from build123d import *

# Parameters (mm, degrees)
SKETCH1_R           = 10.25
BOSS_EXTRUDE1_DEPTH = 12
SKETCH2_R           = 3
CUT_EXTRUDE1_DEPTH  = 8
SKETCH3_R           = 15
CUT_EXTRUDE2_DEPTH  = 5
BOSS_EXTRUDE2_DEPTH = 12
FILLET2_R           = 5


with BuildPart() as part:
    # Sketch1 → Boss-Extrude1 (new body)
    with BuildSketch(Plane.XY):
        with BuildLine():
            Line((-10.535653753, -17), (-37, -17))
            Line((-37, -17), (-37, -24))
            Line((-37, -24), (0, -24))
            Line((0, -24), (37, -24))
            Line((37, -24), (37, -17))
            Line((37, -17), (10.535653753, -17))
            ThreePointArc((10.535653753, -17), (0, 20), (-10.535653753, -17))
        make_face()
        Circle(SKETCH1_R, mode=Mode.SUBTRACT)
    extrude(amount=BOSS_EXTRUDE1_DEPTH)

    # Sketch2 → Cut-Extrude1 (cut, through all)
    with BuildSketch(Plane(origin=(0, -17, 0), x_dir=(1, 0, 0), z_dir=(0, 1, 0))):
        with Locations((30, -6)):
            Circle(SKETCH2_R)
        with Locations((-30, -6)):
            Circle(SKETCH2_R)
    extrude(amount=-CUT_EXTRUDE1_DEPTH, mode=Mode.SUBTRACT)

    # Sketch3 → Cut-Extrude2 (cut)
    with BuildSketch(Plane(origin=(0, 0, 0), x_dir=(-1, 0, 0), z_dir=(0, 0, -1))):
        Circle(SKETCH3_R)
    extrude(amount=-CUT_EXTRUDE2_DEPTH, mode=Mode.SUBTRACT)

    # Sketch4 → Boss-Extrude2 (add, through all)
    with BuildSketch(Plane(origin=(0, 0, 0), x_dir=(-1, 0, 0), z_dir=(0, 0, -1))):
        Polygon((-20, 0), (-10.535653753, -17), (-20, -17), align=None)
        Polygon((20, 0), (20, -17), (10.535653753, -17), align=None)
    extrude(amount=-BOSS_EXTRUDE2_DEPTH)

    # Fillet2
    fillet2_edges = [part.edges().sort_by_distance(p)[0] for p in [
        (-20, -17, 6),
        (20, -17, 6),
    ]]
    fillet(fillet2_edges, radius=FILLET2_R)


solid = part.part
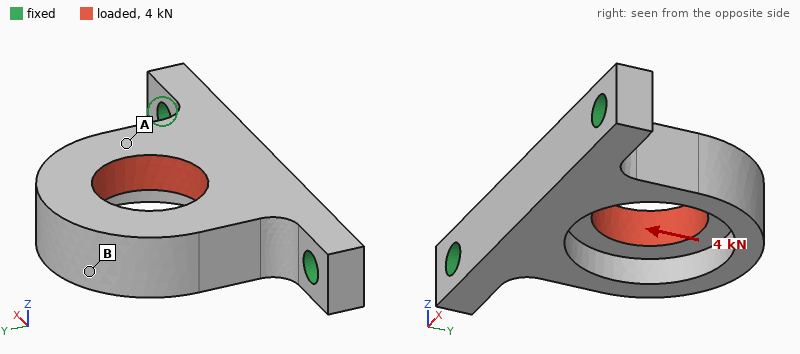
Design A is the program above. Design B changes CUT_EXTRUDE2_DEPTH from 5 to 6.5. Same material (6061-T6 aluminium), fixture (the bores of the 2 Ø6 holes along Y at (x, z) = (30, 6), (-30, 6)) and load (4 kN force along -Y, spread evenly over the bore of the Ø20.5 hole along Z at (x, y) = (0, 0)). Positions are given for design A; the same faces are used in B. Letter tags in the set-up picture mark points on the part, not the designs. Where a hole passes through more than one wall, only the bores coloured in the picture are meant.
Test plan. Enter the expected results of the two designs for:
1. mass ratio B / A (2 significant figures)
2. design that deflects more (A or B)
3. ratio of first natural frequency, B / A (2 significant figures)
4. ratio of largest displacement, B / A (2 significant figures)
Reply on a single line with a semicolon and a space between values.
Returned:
0.96; B; 1.0; 1.3
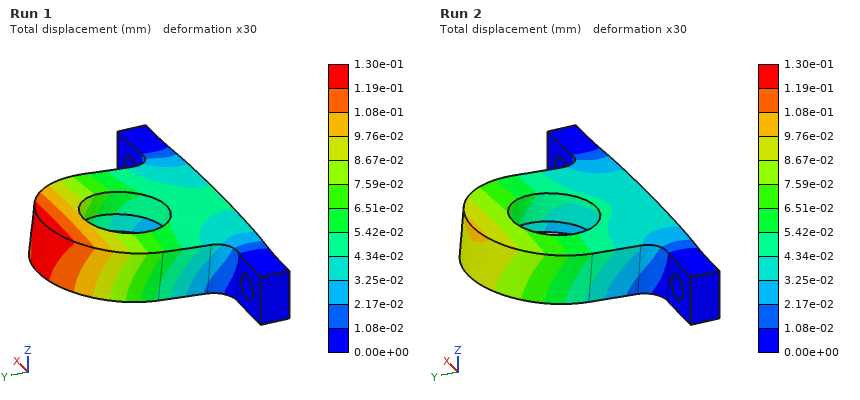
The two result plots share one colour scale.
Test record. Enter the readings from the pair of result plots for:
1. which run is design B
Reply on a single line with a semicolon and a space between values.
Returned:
Run 1
